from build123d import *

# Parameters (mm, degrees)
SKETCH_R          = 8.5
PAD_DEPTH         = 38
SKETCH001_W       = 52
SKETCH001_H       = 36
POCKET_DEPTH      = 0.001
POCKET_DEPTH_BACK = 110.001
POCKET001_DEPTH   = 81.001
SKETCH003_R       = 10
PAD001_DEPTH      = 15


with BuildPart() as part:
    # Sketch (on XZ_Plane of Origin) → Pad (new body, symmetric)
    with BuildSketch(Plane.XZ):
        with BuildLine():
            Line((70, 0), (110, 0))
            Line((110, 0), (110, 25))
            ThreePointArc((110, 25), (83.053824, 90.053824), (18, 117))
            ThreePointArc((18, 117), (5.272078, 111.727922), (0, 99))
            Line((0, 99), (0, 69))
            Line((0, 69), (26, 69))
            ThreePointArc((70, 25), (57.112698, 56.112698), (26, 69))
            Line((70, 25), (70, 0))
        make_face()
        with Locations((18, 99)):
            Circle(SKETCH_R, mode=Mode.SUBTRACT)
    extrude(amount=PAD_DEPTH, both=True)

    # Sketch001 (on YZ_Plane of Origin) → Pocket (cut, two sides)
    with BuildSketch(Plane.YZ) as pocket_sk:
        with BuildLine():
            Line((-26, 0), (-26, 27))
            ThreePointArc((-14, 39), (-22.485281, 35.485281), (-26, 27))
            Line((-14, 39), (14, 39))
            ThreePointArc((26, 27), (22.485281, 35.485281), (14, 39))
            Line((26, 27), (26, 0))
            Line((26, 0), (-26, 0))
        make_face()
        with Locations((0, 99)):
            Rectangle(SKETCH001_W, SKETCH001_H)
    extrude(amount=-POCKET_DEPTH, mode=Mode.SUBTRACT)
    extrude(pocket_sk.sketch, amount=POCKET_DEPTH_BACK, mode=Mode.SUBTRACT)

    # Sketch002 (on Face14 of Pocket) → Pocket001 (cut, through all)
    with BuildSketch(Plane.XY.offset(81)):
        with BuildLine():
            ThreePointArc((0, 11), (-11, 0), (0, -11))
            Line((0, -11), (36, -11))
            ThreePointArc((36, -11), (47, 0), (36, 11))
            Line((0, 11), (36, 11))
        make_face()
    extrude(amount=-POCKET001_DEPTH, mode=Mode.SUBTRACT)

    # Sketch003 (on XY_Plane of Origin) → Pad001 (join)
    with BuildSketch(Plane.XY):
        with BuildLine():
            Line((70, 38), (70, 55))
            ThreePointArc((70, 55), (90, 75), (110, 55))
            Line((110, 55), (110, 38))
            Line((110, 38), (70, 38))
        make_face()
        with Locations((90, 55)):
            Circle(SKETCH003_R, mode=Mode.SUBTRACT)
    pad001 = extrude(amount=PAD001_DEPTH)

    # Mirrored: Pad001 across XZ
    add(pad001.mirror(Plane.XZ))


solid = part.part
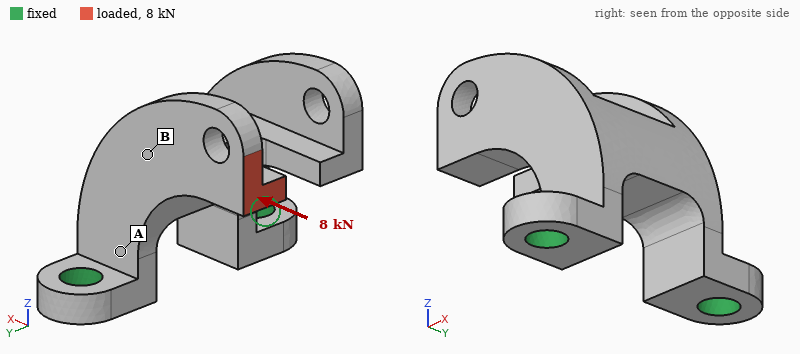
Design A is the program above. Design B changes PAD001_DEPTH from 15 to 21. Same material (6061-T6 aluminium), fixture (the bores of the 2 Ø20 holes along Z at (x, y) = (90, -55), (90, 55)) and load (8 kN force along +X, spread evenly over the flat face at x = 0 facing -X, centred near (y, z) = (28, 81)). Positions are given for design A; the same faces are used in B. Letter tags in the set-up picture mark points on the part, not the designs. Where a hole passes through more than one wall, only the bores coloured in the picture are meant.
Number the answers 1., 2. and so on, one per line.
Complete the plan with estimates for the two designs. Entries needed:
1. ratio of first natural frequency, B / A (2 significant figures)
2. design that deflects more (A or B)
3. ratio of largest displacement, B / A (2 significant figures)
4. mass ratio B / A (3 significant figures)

1. 1.3
2. A
3. 0.64
4. 1.04
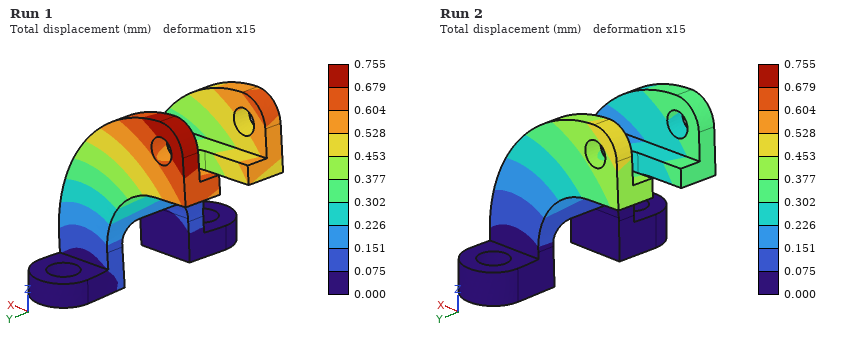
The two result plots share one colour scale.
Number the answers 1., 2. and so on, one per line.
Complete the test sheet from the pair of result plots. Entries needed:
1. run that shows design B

1. Run 2
